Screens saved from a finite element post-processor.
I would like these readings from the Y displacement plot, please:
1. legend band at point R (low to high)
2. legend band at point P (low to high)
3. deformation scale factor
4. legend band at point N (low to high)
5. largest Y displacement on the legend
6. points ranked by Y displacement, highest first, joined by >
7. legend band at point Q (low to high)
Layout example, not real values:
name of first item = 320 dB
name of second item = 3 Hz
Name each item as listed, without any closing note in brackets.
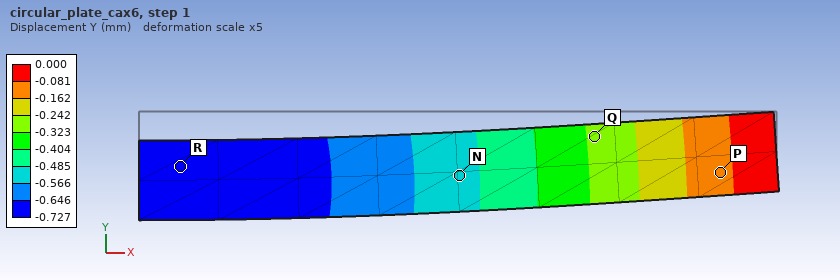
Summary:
legend band at point R = -0.727 to -0.646 mm
legend band at point P = -0.162 to -0.081 mm
deformation scale factor = 5
legend band at point N = -0.566 to -0.485 mm
largest Y displacement on the legend = 0.000 mm
points ranked by Y displacement, highest first, joined by > = P > Q > N > R
legend band at point Q = -0.323 to -0.242 mm
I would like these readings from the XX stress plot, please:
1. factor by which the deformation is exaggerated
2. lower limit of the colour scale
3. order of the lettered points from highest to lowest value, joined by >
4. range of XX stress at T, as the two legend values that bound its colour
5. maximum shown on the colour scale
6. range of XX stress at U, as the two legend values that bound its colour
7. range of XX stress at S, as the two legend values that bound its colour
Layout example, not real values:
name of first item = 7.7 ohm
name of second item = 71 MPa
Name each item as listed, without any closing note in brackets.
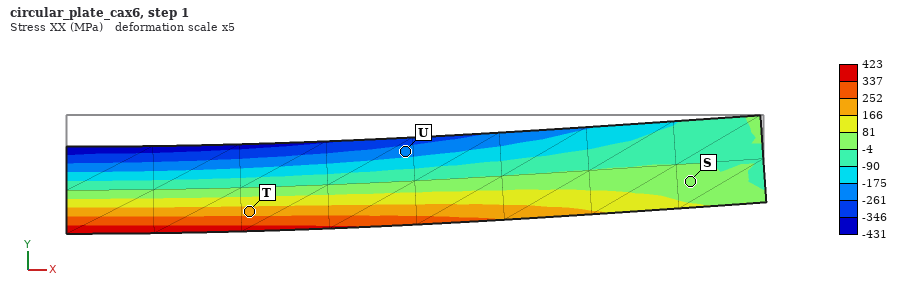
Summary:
factor by which the deformation is exaggerated = 5
lower limit of the colour scale = -431 MPa
order of the lettered points from highest to lowest value, joined by > = T > S > U
range of XX stress at T, as the two legend values that bound its colour = 166 to 252 MPa
maximum shown on the colour scale = 423 MPa
range of XX stress at U, as the two legend values that bound its colour = -261 to -175 MPa
range of XX stress at S, as the two legend values that bound its colour = -4 to 81 MPa
